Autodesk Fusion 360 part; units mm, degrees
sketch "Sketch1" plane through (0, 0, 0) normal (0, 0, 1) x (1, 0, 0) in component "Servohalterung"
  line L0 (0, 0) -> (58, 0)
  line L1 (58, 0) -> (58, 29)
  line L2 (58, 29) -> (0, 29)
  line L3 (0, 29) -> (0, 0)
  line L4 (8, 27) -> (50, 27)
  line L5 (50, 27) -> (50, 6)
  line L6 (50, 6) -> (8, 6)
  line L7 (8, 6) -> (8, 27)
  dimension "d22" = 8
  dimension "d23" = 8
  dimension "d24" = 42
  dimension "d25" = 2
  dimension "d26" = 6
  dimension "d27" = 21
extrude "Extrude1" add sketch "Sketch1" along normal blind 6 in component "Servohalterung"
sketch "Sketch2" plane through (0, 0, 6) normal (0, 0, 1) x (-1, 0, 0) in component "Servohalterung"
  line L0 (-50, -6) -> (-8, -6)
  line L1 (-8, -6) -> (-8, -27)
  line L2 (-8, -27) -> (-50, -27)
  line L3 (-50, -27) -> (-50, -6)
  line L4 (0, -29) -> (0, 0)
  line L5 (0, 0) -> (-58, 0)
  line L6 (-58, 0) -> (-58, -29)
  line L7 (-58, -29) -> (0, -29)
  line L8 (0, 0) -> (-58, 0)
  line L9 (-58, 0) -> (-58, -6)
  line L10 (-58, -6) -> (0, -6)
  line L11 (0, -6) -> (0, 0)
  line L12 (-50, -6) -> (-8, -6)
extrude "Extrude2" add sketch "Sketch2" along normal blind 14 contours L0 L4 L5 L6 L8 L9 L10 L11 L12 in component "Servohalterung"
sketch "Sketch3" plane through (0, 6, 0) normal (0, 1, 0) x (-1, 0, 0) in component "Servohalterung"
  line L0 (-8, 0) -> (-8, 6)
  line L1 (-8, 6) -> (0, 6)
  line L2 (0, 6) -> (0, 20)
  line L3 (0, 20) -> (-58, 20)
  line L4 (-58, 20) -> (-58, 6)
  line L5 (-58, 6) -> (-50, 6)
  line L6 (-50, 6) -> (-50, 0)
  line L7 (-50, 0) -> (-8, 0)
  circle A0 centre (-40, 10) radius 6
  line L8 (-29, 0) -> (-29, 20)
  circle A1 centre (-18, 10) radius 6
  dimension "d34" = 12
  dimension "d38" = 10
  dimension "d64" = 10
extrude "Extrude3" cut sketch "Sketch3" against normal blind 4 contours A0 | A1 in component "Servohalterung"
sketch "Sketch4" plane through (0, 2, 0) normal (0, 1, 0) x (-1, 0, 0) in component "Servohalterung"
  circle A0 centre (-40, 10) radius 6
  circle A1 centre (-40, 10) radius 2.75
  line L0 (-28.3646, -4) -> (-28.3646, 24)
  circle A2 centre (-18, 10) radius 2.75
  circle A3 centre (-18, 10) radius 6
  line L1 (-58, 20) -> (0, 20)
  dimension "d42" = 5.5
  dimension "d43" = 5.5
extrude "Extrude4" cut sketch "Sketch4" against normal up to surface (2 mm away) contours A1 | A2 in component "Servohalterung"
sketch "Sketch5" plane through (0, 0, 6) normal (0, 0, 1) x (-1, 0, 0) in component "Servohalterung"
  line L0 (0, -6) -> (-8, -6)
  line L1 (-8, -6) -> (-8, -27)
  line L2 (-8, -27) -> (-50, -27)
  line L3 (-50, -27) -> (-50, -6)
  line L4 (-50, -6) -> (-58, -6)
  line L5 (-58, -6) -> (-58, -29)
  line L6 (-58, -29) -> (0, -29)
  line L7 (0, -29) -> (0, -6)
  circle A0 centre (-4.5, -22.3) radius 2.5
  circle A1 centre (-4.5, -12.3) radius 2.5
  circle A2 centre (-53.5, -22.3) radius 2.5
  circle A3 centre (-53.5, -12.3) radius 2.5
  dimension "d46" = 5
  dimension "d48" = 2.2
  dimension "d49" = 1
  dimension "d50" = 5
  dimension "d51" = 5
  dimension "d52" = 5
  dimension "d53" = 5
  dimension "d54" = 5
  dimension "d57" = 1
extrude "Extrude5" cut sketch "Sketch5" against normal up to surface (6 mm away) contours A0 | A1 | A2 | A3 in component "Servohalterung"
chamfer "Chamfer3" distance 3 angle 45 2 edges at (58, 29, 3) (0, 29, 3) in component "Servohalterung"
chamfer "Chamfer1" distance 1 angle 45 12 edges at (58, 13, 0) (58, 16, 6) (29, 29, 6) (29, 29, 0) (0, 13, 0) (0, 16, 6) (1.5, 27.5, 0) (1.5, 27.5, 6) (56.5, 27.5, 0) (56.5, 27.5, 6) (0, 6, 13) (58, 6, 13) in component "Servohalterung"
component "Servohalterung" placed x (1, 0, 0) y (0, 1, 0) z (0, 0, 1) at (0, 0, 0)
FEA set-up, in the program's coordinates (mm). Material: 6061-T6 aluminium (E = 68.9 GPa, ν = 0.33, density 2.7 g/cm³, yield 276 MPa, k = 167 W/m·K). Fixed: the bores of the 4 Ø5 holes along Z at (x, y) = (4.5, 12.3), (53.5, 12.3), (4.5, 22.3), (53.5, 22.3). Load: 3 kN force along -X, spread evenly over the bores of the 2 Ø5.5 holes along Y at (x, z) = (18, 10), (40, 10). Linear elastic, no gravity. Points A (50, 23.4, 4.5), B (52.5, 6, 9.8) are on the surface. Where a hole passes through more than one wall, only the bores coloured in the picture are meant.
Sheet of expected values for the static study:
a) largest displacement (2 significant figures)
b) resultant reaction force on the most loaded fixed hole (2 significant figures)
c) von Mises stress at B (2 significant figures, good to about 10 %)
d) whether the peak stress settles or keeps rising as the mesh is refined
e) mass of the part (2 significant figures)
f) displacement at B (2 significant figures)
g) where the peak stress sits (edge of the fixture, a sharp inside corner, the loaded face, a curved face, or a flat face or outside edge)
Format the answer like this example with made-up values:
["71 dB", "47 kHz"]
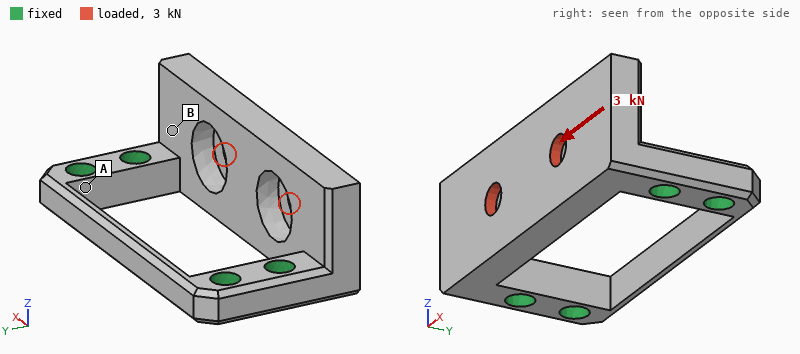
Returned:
["35 µm", "1.6 kN", "29 MPa", "keeps rising", "22 g", "21 µm", "edge of the fixture"]
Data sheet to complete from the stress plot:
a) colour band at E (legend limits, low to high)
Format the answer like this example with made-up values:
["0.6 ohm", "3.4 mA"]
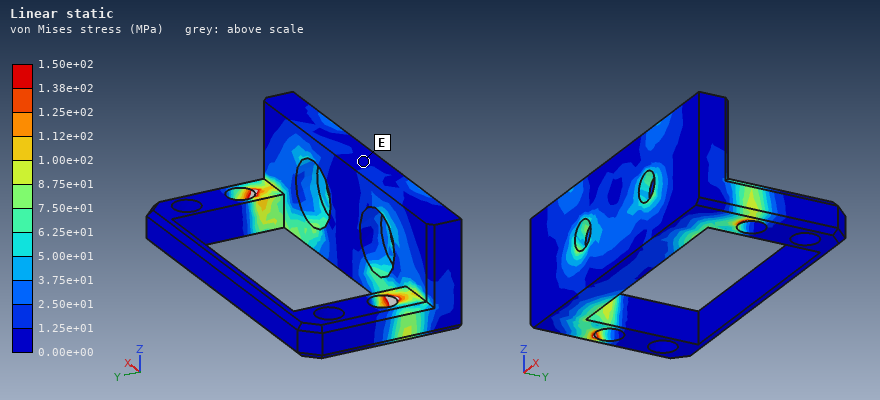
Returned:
["0.00e+00 to 1.25e+01 MPa"]
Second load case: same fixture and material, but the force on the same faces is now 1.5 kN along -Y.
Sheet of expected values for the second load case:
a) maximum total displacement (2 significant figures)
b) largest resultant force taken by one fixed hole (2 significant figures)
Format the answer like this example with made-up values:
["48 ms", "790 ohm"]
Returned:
["0.14 mm", "980 N"]
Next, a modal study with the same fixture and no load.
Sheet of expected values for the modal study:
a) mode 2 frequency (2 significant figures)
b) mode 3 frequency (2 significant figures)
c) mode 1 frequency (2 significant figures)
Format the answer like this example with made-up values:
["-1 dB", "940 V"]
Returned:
["5300 Hz", "10 kHz", "5200 Hz"]
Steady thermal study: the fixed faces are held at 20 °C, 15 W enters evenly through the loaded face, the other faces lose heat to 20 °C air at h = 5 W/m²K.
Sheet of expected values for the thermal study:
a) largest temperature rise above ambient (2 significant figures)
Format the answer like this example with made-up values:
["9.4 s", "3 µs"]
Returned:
["17 K"]
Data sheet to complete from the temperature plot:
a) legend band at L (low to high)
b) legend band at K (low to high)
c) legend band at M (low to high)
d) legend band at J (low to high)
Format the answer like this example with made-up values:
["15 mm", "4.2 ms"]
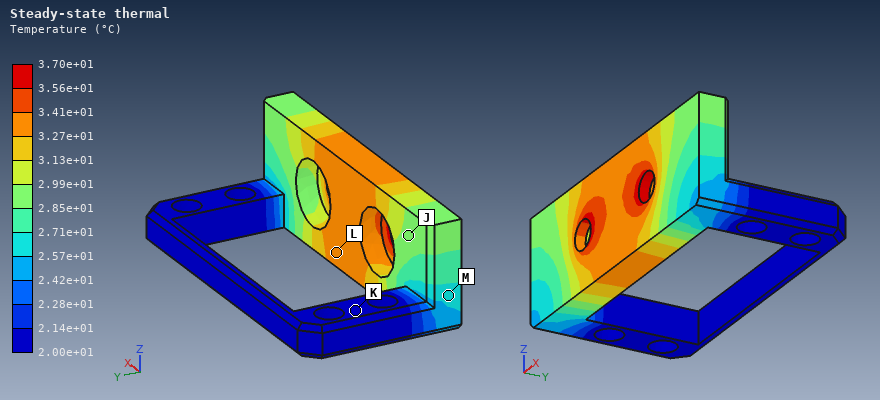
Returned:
["3.27e+01 to 3.41e+01 °C", "2.00e+01 to 2.14e+01 °C", "2.57e+01 to 2.71e+01 °C", "2.85e+01 to 2.99e+01 °C"]
